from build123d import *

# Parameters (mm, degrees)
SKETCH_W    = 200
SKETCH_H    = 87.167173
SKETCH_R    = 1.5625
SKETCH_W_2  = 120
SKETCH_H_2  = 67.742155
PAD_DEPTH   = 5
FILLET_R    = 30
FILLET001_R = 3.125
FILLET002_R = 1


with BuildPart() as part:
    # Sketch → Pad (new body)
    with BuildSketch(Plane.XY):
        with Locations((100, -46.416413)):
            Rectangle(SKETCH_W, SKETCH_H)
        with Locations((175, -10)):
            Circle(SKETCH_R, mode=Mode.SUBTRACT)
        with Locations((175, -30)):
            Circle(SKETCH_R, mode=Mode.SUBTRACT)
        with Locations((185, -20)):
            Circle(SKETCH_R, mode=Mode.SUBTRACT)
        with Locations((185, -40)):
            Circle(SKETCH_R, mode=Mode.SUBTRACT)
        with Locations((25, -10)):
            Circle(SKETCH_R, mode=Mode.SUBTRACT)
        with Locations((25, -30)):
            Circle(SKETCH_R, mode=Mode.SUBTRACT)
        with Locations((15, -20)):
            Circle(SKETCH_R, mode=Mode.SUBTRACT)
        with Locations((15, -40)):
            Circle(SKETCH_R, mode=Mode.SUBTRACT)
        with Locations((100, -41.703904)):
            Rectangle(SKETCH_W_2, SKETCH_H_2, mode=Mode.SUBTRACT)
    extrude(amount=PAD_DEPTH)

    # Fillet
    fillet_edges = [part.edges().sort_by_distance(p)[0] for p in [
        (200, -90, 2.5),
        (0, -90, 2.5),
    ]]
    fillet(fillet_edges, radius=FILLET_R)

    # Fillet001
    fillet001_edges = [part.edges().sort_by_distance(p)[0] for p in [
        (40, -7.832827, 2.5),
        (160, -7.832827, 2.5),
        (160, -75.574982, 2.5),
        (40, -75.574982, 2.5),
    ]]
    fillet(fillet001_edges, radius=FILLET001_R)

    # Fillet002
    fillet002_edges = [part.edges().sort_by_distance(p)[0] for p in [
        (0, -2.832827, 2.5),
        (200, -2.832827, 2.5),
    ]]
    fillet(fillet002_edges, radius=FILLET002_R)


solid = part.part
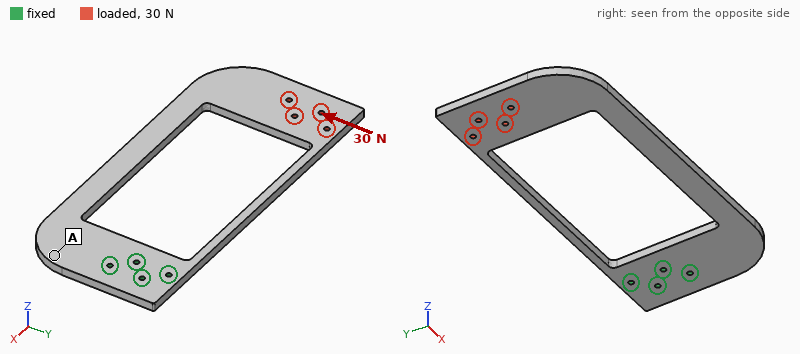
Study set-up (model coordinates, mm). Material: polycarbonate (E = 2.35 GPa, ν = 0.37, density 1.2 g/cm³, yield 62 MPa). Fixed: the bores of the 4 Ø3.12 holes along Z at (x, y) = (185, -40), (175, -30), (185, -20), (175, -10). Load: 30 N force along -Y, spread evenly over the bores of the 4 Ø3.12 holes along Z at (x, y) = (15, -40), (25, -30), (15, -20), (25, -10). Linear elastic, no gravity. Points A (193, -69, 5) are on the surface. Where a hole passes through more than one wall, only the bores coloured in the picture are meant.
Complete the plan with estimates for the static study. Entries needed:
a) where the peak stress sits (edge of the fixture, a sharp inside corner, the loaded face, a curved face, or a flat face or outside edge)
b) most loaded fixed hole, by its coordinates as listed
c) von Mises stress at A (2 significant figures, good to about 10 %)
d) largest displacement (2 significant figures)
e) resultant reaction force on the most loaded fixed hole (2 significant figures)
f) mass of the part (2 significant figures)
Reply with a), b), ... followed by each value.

a) a curved face
b) (185, -40)
c) 1.4 MPa
d) 2.6 mm
e) 130 N
f) 53 g
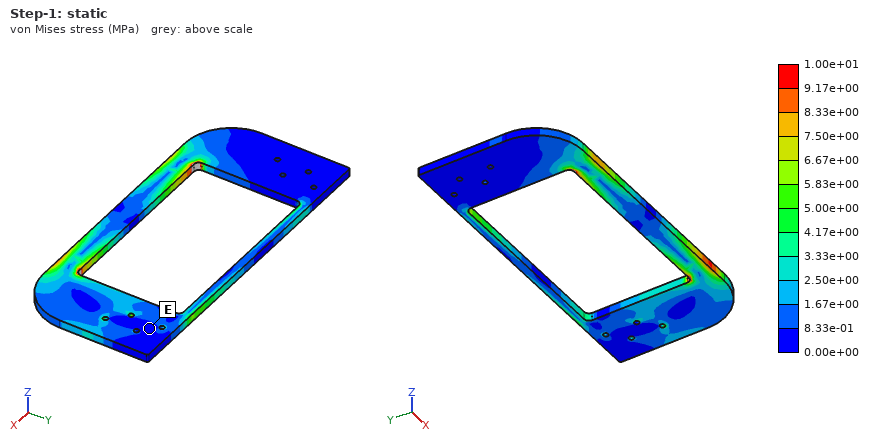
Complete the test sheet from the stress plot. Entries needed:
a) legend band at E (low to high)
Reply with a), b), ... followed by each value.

a) 0.00e+00 to 8.33e-01 MPa
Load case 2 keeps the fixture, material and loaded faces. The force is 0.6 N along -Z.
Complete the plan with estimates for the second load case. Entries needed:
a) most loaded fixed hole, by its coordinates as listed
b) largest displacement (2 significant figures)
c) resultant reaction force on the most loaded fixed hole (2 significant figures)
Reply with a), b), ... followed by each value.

a) (175, -30)
b) 2.0 mm
c) 2.8 N
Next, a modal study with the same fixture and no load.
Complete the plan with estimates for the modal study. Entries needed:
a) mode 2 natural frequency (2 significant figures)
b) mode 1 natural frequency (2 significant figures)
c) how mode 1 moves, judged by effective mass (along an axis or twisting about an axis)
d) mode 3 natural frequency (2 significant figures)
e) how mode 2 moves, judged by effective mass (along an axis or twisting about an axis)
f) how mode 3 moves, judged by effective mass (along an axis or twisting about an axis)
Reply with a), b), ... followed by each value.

a) 81 Hz
b) 21 Hz
c) along Z
d) 110 Hz
e) twisting about X
f) along Y
